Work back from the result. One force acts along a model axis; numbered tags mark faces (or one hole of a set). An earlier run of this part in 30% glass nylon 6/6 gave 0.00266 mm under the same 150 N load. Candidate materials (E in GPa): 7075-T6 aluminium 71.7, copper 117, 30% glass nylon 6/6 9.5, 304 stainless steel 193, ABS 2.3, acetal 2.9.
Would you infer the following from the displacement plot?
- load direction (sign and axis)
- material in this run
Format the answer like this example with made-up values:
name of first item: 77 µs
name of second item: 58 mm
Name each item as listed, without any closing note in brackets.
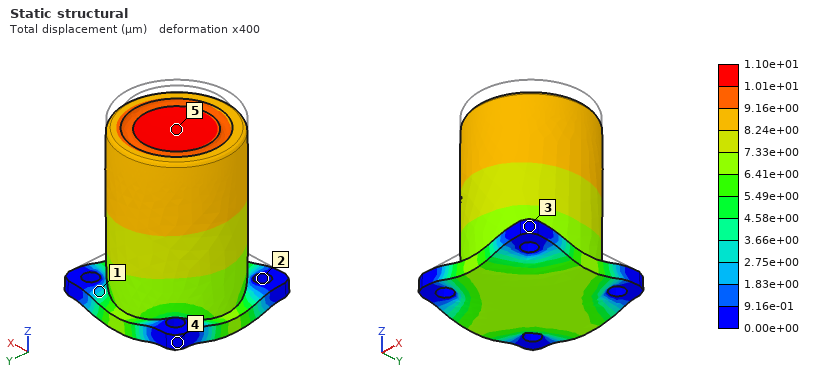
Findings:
load direction: -Z
material in this run: ABS
